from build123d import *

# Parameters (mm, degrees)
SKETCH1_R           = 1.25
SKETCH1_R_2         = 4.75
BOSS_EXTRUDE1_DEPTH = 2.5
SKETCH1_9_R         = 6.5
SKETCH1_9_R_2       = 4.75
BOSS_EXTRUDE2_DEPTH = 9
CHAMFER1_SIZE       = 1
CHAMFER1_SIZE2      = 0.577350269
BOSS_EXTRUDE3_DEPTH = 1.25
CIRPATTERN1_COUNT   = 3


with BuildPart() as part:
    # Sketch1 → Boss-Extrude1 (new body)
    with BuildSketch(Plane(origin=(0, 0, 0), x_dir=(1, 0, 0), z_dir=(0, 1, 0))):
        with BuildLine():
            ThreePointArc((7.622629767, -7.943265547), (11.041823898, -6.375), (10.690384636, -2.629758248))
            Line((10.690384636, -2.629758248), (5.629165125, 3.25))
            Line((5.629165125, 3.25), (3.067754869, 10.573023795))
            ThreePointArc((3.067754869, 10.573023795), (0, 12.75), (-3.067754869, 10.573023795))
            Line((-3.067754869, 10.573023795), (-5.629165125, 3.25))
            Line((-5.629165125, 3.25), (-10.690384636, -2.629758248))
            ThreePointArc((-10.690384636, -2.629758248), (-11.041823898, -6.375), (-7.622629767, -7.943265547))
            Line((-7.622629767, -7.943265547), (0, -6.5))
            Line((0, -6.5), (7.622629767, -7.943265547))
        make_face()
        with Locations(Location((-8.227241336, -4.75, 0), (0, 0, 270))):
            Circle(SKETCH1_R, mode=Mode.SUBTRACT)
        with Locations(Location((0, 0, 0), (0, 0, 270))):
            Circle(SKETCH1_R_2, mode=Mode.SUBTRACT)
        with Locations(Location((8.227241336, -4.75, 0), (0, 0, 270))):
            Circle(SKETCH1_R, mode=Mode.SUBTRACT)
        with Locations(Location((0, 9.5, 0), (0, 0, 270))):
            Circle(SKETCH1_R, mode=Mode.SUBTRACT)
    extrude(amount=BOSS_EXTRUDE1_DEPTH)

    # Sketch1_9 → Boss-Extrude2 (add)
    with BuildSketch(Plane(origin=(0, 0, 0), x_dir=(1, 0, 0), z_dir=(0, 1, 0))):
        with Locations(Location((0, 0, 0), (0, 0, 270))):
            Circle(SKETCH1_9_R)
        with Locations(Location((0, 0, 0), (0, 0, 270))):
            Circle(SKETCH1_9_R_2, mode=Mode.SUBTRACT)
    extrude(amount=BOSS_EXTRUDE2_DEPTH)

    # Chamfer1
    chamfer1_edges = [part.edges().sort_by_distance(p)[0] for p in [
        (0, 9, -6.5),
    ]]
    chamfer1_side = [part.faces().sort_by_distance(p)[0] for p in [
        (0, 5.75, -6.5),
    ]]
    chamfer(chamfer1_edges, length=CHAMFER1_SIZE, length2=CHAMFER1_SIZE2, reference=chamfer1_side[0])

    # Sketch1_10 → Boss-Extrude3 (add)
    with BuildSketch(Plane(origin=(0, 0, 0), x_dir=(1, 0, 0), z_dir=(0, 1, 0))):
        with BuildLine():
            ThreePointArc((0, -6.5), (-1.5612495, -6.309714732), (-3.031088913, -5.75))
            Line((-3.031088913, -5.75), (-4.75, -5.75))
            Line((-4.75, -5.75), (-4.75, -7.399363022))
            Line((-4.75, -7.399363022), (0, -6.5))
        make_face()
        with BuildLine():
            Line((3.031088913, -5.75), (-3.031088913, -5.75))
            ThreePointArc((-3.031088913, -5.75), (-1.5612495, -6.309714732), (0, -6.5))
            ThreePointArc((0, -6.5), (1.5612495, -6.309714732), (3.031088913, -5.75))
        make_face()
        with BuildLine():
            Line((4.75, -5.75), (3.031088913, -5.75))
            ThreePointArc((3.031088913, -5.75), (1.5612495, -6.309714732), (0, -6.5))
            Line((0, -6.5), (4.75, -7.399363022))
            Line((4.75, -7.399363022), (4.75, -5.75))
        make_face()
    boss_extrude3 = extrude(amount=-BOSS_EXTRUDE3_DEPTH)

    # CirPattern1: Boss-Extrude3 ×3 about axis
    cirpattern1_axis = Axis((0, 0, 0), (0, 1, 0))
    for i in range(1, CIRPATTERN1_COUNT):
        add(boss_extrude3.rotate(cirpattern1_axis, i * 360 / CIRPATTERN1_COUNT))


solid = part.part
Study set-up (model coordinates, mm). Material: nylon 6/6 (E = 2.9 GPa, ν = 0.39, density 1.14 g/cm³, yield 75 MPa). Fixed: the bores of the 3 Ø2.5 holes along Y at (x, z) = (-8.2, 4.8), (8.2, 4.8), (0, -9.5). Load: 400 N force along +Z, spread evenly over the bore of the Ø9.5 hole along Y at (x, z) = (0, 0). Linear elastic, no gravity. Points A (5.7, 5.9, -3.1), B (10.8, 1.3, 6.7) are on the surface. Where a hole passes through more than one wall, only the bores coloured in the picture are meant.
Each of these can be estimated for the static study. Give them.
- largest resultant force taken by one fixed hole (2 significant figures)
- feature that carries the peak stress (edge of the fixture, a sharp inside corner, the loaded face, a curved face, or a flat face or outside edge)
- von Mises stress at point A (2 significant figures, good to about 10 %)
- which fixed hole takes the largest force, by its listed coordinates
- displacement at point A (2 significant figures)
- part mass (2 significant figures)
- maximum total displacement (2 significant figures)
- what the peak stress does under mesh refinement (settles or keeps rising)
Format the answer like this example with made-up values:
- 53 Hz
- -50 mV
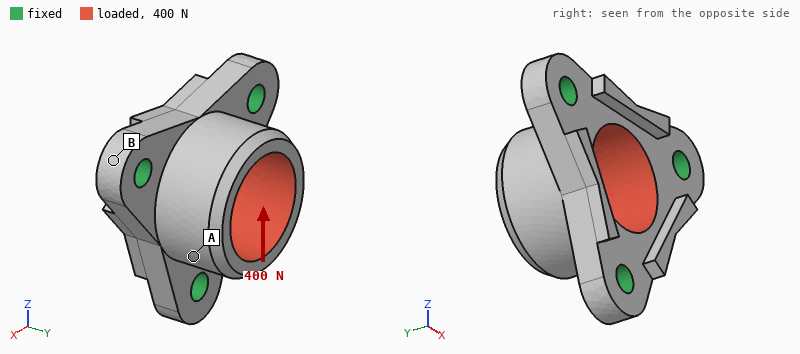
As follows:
- 170 N
- edge of the fixture
- 8.5 MPa
- (0, -9.5)
- 0.081 mm
- 1.0 g
- 0.16 mm
- keeps rising
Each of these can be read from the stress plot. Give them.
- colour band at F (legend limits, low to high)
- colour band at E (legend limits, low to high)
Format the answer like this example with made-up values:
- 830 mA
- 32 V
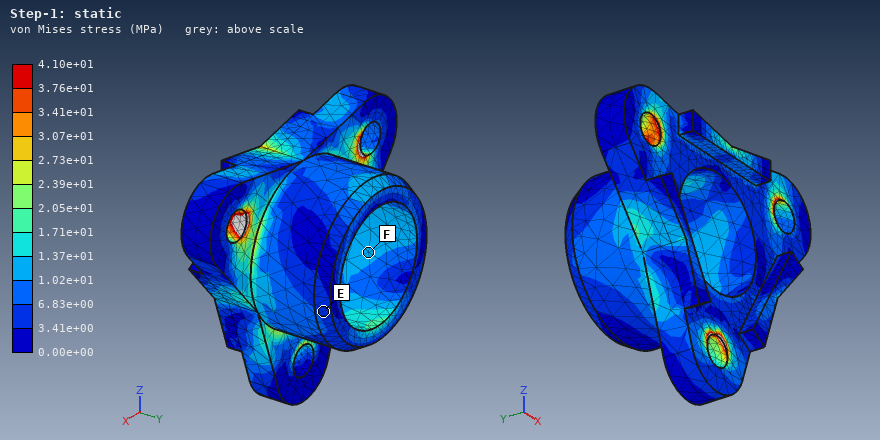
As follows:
- 1.02e+01 to 1.37e+01 MPa
- 3.41e+00 to 6.83e+00 MPa
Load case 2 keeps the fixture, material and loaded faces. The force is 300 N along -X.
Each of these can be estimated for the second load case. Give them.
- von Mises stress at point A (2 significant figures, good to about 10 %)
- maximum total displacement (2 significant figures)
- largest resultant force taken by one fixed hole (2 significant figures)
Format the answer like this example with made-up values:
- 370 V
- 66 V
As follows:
- 6.8 MPa
- 0.11 mm
- 120 N
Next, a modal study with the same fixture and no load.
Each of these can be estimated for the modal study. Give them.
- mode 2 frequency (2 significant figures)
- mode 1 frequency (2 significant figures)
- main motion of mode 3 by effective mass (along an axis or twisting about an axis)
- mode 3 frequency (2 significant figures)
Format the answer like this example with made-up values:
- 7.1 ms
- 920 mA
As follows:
- 12 kHz
- 12 kHz
- along Y
- 15 kHz
